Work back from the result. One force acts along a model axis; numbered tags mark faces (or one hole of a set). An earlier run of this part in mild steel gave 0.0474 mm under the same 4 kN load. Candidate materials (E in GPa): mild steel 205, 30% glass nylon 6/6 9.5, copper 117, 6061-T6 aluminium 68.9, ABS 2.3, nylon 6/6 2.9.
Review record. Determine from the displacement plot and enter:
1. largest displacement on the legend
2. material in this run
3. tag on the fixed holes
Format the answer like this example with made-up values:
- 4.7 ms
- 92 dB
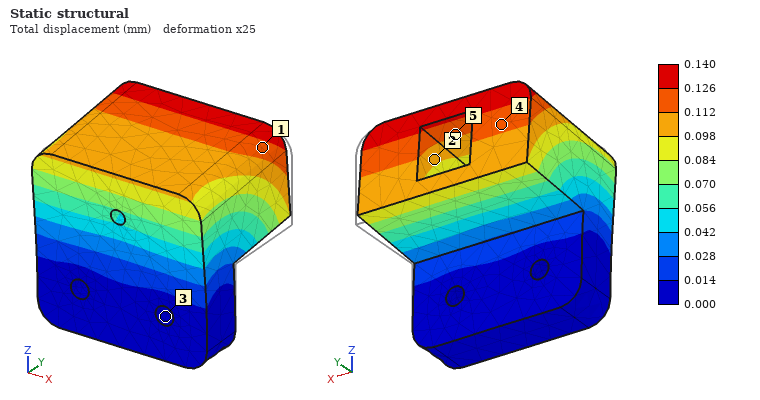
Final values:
- 0.140 mm
- 6061-T6 aluminium
- 3
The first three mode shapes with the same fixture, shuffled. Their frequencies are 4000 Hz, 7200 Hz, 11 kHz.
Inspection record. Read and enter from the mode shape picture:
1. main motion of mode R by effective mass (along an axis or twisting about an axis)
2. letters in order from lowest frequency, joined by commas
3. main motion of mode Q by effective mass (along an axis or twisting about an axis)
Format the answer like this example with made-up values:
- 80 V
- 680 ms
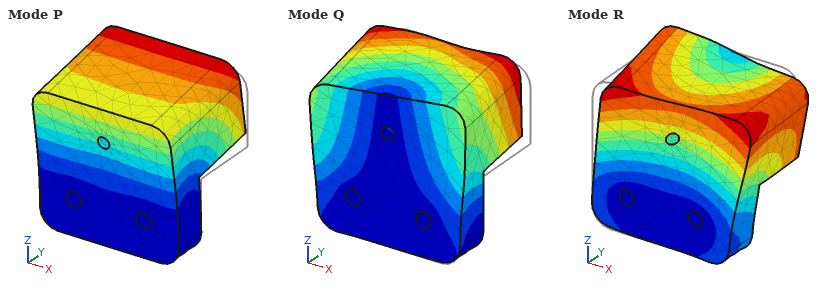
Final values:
- along X
- P, Q, R
- along X
